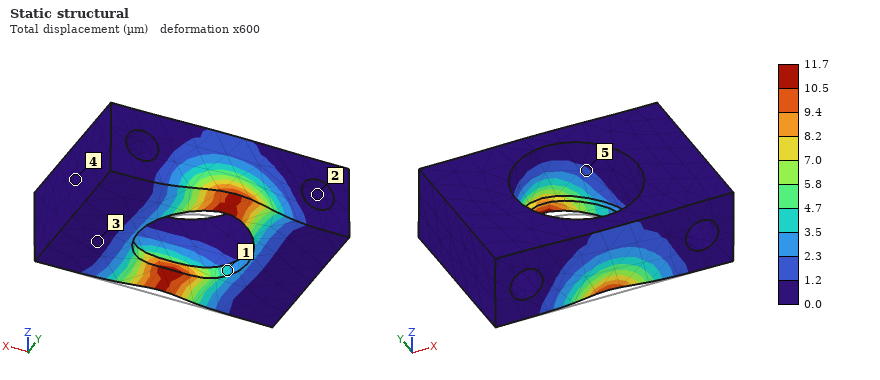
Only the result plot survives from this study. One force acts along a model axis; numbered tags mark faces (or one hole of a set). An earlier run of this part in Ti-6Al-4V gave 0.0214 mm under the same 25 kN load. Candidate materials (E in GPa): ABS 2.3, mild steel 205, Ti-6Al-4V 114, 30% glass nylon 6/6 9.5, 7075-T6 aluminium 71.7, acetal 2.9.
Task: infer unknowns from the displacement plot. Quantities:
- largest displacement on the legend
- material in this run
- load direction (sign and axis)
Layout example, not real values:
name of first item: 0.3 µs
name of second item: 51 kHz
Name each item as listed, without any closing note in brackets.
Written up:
largest displacement on the legend: 11.7 µm
material in this run: mild steel
load direction: +Y
